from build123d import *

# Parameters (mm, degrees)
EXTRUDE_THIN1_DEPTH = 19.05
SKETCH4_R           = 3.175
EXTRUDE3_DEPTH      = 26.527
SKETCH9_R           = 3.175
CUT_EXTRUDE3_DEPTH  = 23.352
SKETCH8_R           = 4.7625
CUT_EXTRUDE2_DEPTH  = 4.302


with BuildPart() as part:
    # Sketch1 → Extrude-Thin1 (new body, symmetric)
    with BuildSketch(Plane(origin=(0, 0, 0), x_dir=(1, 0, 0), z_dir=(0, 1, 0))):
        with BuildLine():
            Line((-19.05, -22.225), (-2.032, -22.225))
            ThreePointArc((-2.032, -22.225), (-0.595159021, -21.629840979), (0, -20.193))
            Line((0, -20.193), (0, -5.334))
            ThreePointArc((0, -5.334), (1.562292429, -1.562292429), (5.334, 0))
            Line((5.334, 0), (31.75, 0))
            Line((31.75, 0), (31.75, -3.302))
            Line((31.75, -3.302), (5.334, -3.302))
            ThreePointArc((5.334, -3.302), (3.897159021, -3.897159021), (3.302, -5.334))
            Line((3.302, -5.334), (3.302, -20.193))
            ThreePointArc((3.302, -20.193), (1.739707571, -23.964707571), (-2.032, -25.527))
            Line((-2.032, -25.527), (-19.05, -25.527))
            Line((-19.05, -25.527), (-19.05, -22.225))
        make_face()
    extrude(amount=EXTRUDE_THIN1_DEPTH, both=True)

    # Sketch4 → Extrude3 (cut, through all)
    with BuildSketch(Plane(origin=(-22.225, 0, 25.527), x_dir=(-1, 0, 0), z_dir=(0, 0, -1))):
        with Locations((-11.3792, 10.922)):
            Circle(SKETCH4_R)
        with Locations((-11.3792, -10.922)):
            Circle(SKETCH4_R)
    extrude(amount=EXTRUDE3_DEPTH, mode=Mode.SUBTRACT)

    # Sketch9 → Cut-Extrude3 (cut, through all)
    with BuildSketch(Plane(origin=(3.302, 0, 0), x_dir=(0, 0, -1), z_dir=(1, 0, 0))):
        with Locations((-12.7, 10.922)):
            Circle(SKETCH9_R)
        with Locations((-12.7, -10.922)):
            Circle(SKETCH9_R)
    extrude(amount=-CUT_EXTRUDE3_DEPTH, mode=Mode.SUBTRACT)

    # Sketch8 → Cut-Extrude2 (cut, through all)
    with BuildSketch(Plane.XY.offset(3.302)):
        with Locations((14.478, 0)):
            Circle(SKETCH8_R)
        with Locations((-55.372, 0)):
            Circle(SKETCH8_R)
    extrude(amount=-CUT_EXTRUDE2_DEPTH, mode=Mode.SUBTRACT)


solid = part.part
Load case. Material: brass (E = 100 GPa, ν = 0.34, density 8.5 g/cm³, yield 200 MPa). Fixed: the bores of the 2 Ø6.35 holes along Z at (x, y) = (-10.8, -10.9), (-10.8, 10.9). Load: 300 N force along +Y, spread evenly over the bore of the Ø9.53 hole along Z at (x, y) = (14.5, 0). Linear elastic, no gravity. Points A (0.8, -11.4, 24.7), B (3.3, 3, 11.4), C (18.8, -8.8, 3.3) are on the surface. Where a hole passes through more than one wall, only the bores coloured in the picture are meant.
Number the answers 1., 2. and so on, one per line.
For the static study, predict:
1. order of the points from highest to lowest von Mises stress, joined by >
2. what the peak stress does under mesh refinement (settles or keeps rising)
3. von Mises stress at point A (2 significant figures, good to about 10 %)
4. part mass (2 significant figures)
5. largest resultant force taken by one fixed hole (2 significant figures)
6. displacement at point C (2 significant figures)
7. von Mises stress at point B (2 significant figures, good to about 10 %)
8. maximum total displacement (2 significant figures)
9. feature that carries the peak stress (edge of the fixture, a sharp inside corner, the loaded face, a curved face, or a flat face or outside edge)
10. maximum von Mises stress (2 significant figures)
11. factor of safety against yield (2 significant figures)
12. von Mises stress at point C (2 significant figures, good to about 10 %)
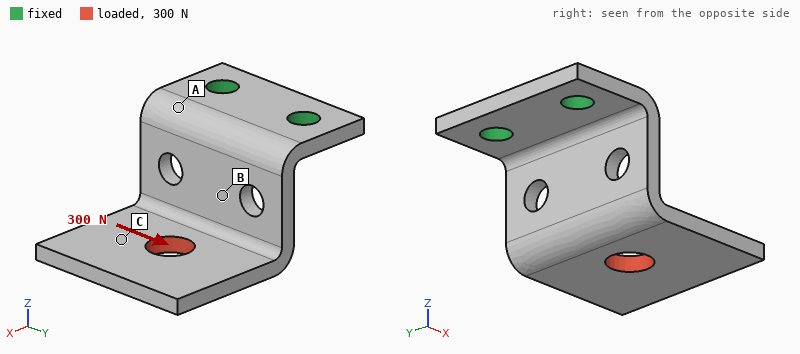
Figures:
1. B > A > C
2. settles
3. 19 MPa
4. 69 g
5. 410 N
6. 59 µm
7. 39 MPa
8. 100 µm
9. a curved face
10. 83 MPa
11. 2.4
12. 7.9 MPa
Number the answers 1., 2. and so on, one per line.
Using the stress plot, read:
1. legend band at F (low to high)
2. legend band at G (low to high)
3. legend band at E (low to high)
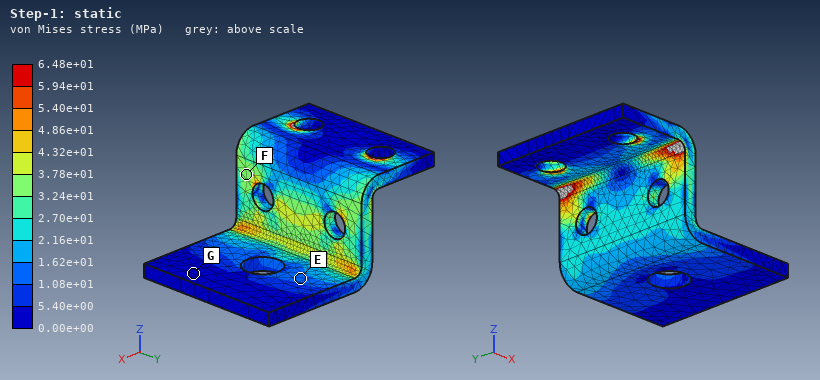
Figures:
1. 3.24e+01 to 3.78e+01 MPa
2. 0.00e+00 to 5.40e+00 MPa
3. 1.08e+01 to 1.62e+01 MPa
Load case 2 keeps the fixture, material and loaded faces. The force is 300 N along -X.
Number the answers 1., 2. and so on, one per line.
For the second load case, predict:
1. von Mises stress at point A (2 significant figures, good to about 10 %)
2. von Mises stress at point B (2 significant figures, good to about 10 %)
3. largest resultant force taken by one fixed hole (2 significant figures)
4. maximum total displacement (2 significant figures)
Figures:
1. 60 MPa
2. 51 MPa
3. 160 N
4. 0.46 mm
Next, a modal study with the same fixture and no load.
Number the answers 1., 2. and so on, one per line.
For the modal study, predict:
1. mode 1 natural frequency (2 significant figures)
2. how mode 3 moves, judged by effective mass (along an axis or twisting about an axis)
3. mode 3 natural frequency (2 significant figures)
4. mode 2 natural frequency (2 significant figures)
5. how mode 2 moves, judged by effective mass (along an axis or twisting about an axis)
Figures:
1. 660 Hz
2. along X
3. 2300 Hz
4. 1500 Hz
5. along Y
